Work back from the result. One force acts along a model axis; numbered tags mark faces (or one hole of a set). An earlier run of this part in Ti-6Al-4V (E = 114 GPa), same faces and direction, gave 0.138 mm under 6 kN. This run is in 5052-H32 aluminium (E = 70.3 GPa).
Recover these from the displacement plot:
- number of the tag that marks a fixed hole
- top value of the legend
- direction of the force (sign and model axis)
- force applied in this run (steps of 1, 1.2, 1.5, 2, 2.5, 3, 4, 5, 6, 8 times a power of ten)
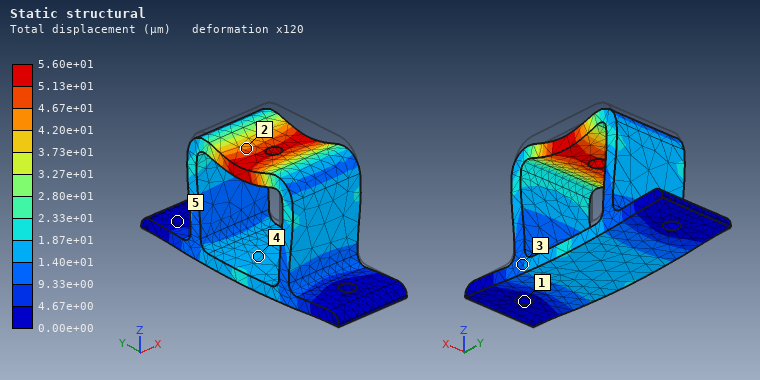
1
5.60e+01 µm
-Z
1.5 kN
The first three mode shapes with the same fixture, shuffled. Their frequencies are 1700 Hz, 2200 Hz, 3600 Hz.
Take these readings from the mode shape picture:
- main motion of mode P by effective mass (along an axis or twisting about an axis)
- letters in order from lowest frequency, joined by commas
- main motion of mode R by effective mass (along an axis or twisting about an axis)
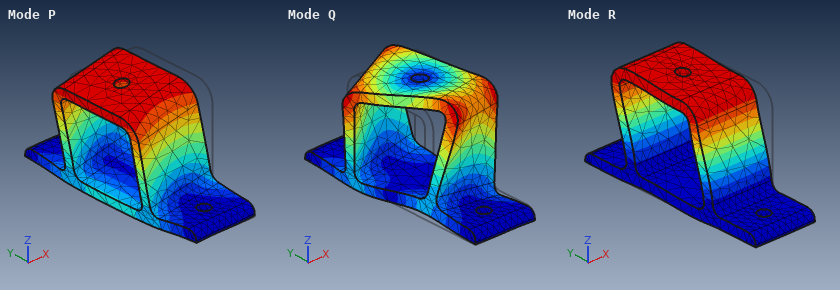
along X
P, R, Q
along Y
